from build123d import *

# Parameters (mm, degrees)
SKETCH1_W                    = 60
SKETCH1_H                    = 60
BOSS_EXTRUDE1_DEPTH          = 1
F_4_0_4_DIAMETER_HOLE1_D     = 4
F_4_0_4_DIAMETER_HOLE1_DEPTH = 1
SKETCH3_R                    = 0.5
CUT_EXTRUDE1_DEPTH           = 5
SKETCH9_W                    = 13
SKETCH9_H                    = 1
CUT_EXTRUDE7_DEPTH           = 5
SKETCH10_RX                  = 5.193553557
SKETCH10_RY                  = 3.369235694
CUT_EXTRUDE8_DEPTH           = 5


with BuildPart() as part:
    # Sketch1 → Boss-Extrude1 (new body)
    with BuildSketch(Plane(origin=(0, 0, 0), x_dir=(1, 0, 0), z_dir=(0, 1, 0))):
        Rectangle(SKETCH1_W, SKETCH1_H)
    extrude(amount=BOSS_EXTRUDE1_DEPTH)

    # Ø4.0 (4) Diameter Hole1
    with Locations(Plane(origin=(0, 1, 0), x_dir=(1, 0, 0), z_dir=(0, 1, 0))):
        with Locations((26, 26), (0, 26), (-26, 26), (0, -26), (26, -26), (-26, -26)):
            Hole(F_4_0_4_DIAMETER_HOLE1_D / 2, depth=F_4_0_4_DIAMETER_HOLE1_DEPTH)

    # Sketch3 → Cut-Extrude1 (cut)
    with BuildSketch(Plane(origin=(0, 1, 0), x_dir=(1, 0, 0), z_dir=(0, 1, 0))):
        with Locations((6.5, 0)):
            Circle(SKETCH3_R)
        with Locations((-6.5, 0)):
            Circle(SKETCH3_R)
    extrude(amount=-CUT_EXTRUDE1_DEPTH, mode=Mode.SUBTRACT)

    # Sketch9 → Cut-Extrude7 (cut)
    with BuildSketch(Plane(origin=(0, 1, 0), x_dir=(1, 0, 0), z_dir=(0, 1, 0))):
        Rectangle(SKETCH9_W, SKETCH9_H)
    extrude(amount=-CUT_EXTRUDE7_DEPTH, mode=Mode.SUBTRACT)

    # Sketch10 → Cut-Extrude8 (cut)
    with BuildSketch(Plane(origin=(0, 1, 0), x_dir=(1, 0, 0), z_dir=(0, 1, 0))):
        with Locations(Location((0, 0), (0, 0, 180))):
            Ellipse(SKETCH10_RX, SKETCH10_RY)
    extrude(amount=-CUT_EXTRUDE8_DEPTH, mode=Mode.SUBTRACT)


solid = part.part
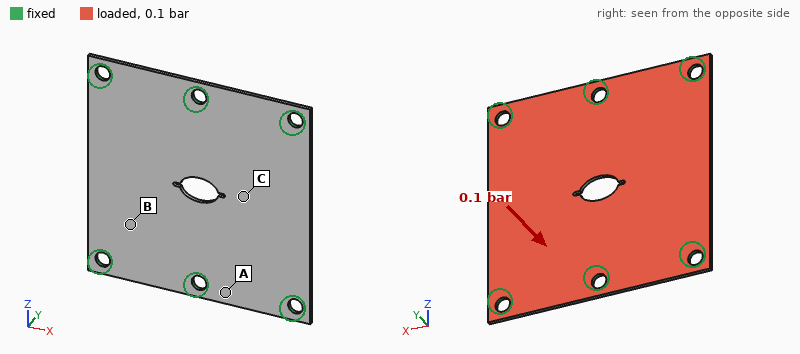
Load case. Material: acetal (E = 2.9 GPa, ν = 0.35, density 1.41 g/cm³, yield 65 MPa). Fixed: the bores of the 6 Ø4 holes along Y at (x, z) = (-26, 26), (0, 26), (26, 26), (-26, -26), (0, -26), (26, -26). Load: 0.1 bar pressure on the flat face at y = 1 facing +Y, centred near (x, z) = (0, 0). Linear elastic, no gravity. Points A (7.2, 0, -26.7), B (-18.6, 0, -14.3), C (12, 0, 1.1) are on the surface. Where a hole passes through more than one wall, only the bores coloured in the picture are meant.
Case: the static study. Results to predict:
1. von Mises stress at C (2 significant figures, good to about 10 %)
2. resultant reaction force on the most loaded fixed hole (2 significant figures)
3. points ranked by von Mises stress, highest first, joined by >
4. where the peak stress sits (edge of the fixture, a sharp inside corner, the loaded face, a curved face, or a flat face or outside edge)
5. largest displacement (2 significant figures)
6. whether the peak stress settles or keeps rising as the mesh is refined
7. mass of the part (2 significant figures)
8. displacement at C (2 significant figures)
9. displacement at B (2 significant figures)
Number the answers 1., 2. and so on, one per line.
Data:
1. 7.1 MPa
2. 7.6 N
3. C > A > B
4. edge of the fixture
5. 0.86 mm
6. keeps rising
7. 4.9 g
8. 0.78 mm
9. 0.38 mm
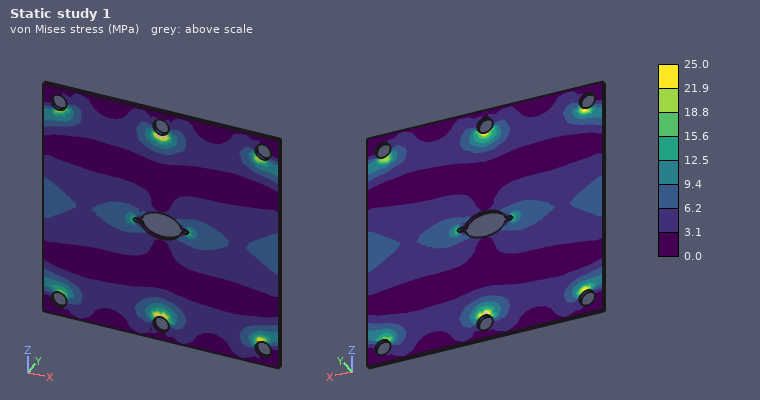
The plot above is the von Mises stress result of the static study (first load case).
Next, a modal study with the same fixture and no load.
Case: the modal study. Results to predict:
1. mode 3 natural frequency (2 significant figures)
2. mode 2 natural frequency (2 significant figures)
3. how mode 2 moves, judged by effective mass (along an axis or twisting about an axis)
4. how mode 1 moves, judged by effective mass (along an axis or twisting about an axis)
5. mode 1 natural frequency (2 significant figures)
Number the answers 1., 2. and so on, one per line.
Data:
1. 1000 Hz
2. 670 Hz
3. twisting about Z
4. along Y
5. 550 Hz
